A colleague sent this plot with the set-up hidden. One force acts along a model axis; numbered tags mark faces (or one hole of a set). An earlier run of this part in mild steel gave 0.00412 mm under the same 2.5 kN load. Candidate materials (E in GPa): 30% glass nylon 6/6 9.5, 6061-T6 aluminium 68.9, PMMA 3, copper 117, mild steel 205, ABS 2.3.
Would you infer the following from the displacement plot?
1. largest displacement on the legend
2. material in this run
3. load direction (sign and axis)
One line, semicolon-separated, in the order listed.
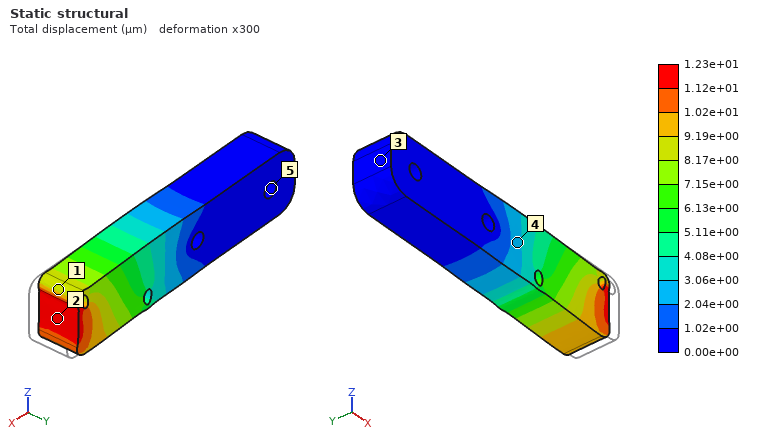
1.23e+01 µm; 6061-T6 aluminium; -X
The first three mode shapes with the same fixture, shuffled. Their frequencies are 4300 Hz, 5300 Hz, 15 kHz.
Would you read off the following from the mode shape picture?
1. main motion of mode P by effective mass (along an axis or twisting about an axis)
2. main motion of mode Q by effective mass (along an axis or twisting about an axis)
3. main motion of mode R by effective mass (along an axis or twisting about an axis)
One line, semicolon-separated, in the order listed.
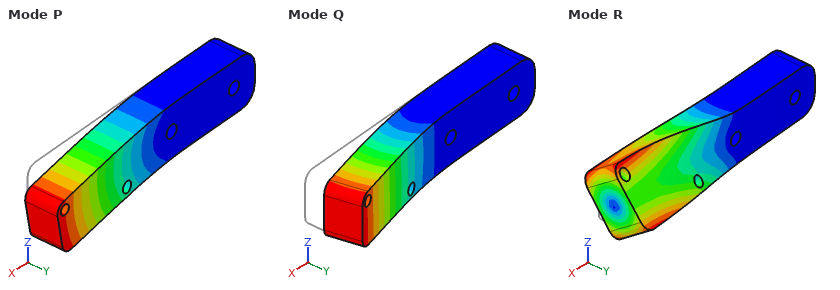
along Z; along Y; twisting about X
